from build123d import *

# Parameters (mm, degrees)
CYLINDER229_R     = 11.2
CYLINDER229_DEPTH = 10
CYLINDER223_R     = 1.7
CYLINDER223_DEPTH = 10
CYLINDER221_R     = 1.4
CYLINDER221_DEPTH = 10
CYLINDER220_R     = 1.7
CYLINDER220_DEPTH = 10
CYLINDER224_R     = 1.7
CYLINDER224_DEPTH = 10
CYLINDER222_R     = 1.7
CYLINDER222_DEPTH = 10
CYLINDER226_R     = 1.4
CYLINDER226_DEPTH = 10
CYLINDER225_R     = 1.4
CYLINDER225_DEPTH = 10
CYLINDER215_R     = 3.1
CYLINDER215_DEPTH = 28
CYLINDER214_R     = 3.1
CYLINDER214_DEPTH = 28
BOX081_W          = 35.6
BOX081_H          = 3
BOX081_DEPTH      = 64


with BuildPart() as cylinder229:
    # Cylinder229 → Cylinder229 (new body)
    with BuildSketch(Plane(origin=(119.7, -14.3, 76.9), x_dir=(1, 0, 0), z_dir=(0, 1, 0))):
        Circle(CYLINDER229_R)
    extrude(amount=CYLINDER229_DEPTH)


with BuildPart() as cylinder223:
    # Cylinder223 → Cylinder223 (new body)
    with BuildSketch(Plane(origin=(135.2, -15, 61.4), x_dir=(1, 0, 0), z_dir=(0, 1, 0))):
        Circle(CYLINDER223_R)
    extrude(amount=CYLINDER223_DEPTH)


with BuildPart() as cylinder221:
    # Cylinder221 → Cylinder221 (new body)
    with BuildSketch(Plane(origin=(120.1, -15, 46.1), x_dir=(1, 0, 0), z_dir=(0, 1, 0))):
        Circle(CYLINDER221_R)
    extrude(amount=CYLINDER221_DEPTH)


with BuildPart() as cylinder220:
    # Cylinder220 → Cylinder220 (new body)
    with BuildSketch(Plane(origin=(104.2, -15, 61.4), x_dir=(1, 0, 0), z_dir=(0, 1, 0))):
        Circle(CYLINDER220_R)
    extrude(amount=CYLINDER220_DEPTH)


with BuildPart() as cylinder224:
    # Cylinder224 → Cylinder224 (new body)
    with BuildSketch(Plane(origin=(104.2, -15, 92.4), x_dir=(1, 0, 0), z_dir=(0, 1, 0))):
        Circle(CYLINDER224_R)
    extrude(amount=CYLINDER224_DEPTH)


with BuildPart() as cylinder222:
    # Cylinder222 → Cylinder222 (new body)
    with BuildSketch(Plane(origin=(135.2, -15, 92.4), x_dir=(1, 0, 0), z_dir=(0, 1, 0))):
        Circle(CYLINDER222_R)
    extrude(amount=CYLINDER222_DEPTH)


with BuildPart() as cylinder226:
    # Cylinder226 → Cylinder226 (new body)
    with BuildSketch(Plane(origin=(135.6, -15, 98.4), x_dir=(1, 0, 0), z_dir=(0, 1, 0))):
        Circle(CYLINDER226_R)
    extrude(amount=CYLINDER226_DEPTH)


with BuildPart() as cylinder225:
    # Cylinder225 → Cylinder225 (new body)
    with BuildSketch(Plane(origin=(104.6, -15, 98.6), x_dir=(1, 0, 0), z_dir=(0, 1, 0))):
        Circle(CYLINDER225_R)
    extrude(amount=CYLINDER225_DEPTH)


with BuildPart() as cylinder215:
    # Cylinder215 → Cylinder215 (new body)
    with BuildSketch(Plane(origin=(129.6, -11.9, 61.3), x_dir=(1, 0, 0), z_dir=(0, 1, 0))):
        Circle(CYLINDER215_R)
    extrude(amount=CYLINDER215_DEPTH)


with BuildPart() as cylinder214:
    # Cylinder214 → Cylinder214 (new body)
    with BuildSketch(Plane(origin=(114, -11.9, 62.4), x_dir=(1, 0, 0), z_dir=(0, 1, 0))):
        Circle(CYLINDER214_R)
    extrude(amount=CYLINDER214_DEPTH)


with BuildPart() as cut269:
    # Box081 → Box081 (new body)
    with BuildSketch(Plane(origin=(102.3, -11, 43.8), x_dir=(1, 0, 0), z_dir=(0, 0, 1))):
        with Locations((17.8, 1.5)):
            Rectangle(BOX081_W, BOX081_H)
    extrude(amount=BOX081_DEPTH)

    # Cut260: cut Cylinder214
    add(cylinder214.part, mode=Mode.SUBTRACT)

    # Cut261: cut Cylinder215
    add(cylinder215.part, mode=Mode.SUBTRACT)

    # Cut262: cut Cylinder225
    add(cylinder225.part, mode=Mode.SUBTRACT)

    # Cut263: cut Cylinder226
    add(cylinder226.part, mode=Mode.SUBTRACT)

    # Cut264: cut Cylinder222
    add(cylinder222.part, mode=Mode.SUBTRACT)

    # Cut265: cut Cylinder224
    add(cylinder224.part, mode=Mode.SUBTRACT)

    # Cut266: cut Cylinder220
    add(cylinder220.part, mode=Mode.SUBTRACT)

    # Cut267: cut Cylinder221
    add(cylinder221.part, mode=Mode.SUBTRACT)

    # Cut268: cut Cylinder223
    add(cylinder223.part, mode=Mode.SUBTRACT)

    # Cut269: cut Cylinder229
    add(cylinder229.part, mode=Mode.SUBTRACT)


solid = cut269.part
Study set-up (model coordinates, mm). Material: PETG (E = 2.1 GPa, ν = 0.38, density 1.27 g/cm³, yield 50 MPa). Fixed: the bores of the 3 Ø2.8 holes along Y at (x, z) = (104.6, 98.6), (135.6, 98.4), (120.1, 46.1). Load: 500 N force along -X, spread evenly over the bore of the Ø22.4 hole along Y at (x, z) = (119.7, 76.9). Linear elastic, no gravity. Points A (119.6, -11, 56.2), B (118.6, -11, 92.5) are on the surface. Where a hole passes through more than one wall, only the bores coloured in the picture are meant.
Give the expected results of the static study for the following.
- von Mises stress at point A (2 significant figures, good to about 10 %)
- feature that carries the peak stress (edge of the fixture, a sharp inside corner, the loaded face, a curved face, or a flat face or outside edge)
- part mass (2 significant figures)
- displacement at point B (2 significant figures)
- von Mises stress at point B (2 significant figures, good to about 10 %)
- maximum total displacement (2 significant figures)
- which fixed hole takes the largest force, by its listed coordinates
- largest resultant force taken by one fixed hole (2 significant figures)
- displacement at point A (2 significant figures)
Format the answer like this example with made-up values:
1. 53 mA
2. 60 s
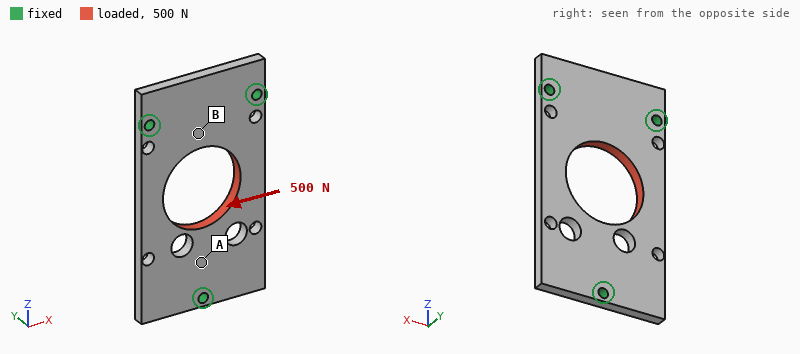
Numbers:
1. 3.1 MPa
2. a curved face
3. 6.7 g
4. 0.047 mm
5. 8.5 MPa
6. 0.22 mm
7. (120.1, 46.1)
8. 190 N
9. 0.096 mm
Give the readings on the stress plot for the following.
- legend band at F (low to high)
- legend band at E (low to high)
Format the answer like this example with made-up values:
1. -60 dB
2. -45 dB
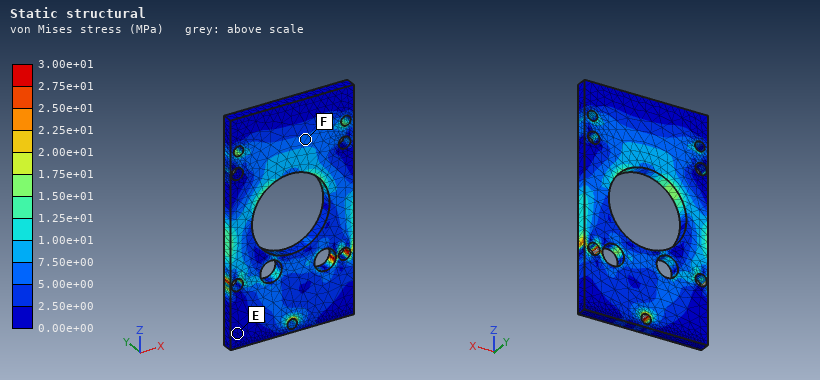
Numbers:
1. 5.00e+00 to 7.50e+00 MPa
2. 0.00e+00 to 2.50e+00 MPa
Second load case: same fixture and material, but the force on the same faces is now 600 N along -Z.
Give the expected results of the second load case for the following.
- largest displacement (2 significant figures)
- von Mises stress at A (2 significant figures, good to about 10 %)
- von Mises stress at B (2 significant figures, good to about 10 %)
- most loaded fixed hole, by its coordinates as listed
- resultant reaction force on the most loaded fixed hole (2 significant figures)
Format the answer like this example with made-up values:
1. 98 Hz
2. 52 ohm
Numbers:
1. 0.10 mm
2. 6.3 MPa
3. 2.4 MPa
4. (120.1, 46.1)
5. 220 N
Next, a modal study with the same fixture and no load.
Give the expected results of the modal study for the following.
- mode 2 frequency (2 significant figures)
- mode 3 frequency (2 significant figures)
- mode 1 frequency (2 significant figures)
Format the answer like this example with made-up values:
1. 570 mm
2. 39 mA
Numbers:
1. 1200 Hz
2. 2400 Hz
3. 1200 Hz
